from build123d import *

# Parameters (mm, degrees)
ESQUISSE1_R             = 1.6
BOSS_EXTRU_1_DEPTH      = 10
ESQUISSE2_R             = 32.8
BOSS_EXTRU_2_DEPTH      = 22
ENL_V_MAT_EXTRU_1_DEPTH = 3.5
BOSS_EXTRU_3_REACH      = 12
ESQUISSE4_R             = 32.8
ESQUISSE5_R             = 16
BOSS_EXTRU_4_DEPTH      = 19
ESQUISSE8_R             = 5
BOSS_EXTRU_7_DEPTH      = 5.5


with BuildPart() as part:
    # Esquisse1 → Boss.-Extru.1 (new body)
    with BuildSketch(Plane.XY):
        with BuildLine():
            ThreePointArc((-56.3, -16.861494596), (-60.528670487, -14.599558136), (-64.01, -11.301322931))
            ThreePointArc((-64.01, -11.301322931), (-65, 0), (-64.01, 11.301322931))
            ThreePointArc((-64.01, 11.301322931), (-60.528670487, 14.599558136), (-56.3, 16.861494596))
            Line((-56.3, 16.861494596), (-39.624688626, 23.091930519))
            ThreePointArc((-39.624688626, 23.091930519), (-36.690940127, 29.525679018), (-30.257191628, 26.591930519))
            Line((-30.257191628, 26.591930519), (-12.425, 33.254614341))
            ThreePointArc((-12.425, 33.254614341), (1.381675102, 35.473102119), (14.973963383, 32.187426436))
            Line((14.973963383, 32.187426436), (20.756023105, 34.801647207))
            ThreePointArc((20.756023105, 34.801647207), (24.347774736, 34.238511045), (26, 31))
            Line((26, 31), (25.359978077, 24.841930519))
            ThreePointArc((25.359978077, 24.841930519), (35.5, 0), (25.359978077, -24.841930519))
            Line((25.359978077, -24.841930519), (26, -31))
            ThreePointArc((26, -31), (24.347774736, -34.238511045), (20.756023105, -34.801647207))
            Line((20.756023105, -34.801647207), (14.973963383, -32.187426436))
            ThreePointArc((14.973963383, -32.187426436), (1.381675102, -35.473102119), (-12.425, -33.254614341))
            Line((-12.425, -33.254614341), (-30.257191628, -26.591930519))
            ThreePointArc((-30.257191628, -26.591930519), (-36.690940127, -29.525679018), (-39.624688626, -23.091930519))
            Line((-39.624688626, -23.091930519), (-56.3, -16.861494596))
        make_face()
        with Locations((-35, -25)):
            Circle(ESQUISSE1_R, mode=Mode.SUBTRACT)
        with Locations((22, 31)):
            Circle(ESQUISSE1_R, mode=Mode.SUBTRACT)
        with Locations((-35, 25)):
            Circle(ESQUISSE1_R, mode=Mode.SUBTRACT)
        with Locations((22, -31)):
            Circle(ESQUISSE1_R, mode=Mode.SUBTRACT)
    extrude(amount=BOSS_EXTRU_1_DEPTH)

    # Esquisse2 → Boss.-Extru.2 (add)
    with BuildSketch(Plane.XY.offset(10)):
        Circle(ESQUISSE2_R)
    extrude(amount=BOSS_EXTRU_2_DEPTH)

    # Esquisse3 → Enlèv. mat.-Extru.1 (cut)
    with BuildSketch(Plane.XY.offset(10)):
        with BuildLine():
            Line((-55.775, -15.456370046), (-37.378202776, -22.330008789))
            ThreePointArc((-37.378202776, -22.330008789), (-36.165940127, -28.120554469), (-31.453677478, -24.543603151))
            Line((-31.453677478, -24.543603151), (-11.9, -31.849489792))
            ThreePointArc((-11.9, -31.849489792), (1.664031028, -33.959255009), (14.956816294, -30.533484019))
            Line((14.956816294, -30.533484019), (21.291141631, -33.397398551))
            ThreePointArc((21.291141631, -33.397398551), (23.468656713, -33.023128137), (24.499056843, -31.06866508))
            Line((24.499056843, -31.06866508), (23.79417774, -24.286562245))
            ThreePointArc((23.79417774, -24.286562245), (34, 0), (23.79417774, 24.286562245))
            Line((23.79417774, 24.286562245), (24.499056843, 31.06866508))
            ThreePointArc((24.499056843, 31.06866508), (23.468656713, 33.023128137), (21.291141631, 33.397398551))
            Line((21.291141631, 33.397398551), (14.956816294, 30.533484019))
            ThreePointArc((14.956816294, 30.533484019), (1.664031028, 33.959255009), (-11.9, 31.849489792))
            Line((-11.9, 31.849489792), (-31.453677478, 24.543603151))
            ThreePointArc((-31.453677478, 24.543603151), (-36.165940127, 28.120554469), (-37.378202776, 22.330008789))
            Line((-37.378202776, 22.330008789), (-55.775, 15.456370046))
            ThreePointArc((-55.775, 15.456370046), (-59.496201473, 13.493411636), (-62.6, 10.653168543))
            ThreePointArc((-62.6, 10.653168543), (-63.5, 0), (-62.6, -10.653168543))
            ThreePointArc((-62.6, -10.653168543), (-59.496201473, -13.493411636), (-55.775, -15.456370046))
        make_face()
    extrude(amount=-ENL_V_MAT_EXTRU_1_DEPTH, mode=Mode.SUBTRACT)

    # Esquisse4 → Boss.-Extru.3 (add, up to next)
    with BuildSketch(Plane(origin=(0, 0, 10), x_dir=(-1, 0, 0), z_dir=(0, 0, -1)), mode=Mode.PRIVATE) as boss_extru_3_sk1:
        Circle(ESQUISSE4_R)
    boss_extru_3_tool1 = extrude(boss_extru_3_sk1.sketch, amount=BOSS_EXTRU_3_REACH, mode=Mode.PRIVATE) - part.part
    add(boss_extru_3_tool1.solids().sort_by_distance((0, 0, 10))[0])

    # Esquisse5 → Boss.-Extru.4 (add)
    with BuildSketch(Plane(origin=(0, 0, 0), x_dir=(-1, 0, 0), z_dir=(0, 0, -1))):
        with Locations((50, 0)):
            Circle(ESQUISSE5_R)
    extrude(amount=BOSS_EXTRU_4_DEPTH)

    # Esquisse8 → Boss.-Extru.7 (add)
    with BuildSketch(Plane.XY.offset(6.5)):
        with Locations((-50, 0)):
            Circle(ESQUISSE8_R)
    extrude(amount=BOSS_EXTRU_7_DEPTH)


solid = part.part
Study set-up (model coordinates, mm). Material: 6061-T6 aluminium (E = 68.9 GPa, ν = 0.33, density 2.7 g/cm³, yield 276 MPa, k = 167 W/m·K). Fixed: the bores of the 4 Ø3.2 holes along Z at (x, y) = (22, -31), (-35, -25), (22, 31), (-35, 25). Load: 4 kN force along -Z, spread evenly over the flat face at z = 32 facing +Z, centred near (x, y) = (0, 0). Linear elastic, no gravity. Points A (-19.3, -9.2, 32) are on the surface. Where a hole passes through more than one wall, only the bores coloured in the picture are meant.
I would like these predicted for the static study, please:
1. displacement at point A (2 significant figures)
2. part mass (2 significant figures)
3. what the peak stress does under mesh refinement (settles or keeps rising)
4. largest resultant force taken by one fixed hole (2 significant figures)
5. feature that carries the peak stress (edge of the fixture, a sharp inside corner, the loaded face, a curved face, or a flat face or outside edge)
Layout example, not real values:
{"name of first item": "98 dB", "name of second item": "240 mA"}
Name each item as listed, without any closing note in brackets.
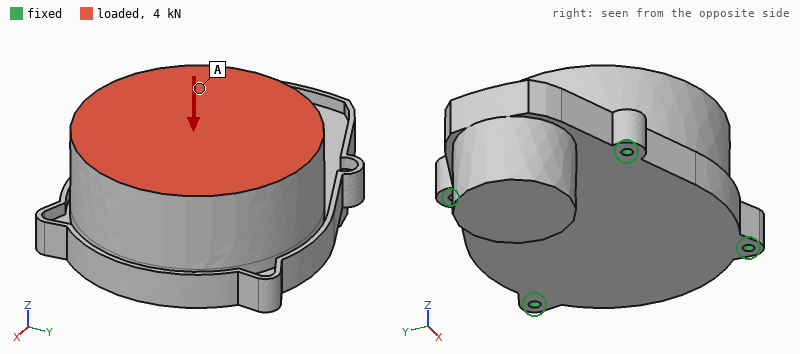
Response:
{"displacement at point A": "9.5 µm", "part mass": "370 g", "what the peak stress does under mesh refinement": "keeps rising", "largest resultant force taken by one fixed hole": "1.3 kN", "feature that carries the peak stress": "edge of the fixture"}
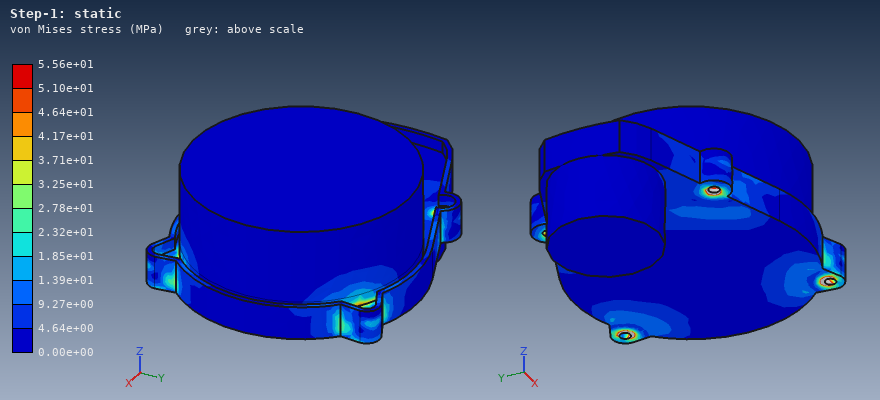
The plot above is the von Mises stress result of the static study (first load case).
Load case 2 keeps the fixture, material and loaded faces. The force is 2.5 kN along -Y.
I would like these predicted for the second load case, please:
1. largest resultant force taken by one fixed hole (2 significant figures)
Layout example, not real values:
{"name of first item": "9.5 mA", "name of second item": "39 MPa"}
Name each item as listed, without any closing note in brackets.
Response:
{"largest resultant force taken by one fixed hole": "1.3 kN"}
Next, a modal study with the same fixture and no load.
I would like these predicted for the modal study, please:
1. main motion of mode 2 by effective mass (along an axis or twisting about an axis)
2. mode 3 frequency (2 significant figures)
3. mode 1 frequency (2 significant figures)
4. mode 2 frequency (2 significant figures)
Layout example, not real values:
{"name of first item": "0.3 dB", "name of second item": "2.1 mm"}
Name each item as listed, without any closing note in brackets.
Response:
{"main motion of mode 2 by effective mass": "along Z", "mode 3 frequency": "6400 Hz", "mode 1 frequency": "2900 Hz", "mode 2 frequency": "5700 Hz"}
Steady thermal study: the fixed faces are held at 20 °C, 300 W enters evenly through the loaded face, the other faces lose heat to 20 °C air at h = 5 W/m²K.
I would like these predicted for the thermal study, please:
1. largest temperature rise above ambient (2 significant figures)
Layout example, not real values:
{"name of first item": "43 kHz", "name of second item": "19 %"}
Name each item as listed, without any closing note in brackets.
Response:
{"largest temperature rise above ambient": "65 K"}
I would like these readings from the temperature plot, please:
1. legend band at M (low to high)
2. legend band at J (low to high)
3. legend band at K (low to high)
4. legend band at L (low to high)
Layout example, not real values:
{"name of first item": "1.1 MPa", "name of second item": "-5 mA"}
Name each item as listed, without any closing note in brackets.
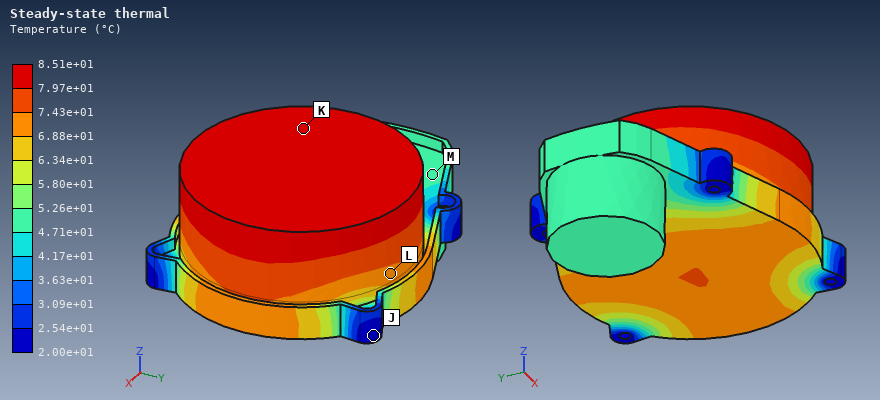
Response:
{"legend band at M": "4.71e+01 to 5.26e+01 °C", "legend band at J": "2.00e+01 to 2.54e+01 °C", "legend band at K": "7.97e+01 to 8.51e+01 °C", "legend band at L": "6.88e+01 to 7.43e+01 °C"}
